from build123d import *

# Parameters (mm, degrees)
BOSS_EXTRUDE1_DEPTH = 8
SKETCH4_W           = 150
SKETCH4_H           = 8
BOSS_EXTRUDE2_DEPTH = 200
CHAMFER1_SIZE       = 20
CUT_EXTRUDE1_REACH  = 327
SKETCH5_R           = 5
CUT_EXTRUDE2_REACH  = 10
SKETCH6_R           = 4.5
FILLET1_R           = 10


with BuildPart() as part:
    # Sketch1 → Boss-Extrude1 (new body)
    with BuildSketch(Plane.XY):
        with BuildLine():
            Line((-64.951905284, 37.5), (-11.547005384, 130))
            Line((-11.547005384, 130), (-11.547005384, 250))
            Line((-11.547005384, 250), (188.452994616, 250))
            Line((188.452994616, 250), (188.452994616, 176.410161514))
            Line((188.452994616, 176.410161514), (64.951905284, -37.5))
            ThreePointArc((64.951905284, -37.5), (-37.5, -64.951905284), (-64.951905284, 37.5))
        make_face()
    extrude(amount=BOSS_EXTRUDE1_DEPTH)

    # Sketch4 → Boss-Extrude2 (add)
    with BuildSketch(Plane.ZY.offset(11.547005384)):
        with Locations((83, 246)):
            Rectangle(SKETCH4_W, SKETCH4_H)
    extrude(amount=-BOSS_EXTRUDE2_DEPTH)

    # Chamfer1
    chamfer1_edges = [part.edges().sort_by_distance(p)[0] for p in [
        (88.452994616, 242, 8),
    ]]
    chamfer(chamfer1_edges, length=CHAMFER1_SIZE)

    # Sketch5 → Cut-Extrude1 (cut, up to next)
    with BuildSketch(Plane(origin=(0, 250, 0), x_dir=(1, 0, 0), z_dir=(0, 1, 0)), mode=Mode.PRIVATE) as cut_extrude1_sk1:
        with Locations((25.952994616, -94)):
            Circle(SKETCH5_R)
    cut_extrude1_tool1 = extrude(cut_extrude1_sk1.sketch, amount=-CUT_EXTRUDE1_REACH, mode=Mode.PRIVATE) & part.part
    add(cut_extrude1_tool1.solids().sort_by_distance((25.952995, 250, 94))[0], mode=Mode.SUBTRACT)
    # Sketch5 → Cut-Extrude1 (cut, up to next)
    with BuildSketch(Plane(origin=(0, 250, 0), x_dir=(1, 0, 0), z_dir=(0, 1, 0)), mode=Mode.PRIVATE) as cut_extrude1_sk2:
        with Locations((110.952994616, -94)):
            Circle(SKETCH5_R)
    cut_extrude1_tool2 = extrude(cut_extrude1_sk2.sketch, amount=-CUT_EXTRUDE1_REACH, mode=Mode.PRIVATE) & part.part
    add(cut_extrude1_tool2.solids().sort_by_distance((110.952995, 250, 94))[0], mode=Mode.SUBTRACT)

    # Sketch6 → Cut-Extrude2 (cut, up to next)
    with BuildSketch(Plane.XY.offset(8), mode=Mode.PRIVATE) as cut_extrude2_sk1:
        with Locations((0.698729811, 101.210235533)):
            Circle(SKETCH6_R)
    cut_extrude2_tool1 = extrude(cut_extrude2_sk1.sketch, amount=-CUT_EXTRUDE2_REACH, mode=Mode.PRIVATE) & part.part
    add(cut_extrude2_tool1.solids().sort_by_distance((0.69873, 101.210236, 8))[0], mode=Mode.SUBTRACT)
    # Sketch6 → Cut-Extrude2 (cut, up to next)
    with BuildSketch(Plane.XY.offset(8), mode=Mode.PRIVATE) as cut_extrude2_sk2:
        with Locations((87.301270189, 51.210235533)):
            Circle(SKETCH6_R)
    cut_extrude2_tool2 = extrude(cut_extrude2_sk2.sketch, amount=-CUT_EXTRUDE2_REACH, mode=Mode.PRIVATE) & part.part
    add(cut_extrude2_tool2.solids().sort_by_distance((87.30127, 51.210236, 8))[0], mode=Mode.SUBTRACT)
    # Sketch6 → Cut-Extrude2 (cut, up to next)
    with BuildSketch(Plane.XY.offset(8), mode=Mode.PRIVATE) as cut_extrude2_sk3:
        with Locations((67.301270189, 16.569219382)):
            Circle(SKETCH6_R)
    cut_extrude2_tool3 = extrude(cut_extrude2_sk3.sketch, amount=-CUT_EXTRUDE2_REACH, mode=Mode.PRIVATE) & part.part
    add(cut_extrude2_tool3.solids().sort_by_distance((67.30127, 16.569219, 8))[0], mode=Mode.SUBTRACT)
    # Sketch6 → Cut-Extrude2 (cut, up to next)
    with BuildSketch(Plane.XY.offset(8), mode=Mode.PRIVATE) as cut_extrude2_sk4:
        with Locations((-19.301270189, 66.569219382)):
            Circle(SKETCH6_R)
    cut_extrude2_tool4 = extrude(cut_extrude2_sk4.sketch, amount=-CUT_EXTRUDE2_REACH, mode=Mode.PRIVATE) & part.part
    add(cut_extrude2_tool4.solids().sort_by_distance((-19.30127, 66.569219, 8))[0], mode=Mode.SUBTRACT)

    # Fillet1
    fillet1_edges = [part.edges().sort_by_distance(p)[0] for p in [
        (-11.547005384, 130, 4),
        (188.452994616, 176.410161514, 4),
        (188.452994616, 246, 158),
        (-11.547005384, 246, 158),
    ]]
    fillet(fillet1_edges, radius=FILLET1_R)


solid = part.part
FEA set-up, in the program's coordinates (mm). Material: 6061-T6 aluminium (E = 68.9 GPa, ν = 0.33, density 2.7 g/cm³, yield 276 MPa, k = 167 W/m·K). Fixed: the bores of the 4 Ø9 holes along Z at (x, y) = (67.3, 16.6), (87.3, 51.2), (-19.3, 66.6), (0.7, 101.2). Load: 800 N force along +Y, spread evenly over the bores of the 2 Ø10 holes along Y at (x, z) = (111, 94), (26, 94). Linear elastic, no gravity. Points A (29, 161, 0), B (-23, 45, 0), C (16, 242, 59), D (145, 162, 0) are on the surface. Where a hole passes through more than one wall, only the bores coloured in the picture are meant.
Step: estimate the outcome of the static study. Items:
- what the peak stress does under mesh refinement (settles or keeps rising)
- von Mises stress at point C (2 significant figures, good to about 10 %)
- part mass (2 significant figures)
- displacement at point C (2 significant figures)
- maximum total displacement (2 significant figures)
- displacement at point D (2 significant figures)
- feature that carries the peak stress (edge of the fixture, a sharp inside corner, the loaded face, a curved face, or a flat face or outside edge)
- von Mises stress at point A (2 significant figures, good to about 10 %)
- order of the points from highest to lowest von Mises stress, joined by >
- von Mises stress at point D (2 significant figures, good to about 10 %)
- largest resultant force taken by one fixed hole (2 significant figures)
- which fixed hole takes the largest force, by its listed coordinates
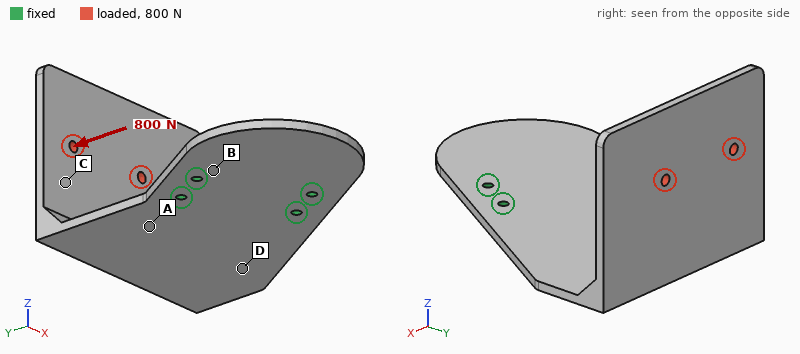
keeps rising
13 MPa
1.9 kg
2.0 mm
4.1 mm
0.76 mm
edge of the fixture
37 MPa
A > D > C > B
29 MPa
770 N
(0.7, 101.2)
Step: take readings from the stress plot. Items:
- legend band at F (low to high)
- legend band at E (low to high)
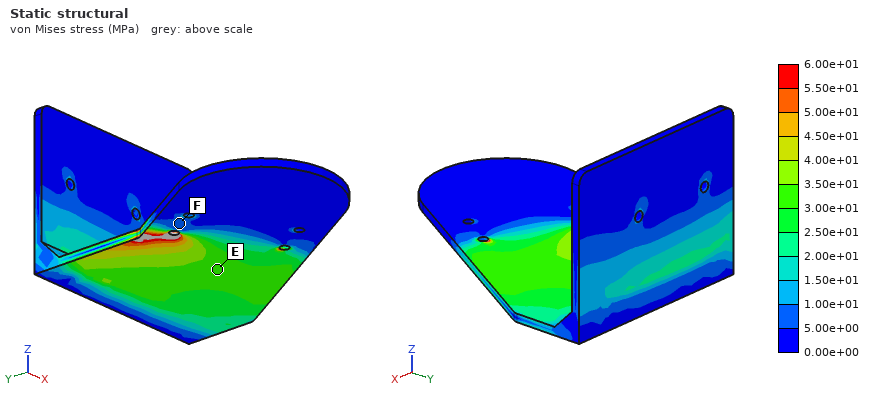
5.00e+00 to 1.00e+01 MPa
3.00e+01 to 3.50e+01 MPa
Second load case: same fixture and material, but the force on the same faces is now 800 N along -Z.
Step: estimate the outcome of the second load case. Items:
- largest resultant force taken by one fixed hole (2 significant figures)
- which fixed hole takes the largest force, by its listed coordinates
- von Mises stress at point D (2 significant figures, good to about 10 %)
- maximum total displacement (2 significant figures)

1.6 kN
(0.7, 101.2)
22 MPa
4.9 mm
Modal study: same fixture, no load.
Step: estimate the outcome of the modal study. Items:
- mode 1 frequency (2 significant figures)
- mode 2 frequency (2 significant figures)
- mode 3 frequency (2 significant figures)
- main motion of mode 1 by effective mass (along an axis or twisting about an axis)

71 Hz
160 Hz
290 Hz
along Z
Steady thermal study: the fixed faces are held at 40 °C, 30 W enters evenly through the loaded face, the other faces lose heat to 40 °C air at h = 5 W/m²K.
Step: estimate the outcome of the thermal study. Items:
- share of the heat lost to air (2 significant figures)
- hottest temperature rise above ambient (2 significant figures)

33 %
26 K
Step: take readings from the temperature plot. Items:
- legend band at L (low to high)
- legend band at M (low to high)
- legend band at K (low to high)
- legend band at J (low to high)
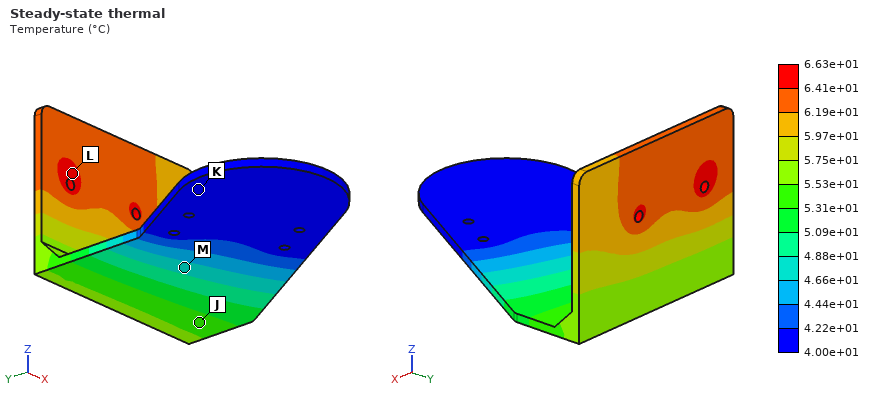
6.41e+01 to 6.63e+01 °C
4.66e+01 to 4.88e+01 °C
4.00e+01 to 4.22e+01 °C
5.31e+01 to 5.53e+01 °C
